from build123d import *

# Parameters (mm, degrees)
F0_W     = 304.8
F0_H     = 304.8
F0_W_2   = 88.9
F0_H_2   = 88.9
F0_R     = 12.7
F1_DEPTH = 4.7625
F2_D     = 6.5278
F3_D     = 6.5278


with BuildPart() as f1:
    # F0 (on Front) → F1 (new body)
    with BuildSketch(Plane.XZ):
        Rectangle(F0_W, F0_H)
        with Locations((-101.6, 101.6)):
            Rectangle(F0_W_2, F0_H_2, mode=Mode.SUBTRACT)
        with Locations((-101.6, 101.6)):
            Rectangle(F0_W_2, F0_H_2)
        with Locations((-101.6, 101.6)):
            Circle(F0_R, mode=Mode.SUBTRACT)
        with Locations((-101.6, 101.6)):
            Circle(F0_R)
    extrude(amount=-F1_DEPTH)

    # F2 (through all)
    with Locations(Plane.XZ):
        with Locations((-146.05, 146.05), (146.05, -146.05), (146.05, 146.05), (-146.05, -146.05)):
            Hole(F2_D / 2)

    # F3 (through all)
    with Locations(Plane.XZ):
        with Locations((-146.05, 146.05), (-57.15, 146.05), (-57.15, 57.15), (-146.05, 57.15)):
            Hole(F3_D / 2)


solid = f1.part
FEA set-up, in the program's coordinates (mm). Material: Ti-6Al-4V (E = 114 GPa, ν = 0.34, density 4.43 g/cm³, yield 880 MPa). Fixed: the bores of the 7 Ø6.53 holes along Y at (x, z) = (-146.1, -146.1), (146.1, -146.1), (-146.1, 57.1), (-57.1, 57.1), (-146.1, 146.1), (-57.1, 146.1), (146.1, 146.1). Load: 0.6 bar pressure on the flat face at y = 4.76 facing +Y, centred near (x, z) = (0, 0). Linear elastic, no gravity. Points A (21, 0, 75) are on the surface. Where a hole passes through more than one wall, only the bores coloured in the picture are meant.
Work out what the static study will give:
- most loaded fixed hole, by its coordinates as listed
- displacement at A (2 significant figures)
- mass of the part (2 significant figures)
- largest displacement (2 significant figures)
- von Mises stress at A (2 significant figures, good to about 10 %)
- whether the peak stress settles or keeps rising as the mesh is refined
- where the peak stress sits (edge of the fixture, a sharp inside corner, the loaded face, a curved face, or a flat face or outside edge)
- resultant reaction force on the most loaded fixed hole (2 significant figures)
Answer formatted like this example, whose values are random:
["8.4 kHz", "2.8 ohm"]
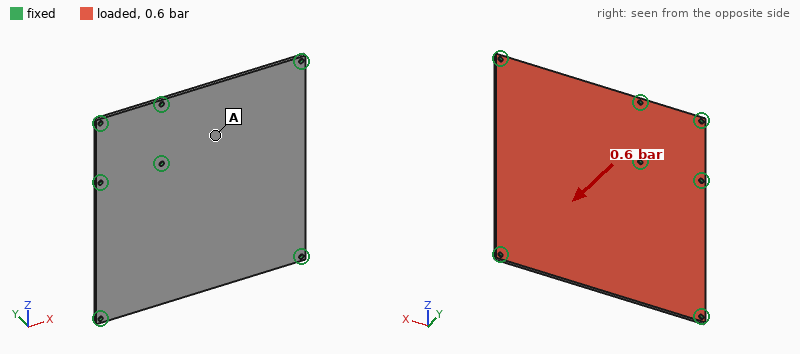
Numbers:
["(-57.1, 57.1)", "0.64 mm", "2.0 kg", "1.6 mm", "36 MPa", "keeps rising", "edge of the fixture", "2.4 kN"]
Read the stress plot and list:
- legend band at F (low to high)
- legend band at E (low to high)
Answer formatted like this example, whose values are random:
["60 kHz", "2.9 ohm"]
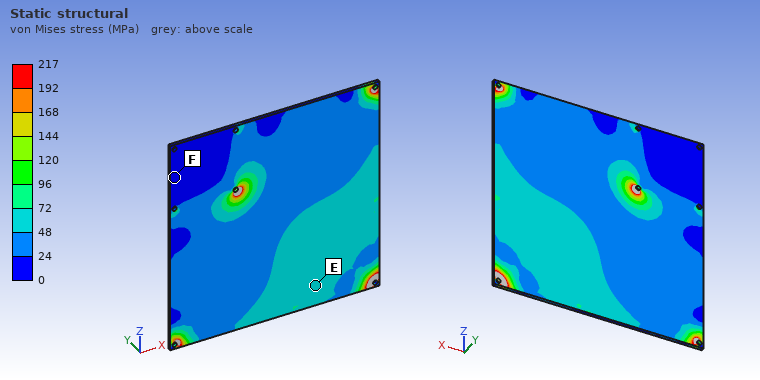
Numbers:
["0 to 24 MPa", "48 to 72 MPa"]
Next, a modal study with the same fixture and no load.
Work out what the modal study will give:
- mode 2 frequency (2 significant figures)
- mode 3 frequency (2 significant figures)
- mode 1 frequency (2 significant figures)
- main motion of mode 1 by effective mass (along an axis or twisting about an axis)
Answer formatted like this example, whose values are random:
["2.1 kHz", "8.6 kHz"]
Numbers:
["320 Hz", "560 Hz", "250 Hz", "along Y"]
